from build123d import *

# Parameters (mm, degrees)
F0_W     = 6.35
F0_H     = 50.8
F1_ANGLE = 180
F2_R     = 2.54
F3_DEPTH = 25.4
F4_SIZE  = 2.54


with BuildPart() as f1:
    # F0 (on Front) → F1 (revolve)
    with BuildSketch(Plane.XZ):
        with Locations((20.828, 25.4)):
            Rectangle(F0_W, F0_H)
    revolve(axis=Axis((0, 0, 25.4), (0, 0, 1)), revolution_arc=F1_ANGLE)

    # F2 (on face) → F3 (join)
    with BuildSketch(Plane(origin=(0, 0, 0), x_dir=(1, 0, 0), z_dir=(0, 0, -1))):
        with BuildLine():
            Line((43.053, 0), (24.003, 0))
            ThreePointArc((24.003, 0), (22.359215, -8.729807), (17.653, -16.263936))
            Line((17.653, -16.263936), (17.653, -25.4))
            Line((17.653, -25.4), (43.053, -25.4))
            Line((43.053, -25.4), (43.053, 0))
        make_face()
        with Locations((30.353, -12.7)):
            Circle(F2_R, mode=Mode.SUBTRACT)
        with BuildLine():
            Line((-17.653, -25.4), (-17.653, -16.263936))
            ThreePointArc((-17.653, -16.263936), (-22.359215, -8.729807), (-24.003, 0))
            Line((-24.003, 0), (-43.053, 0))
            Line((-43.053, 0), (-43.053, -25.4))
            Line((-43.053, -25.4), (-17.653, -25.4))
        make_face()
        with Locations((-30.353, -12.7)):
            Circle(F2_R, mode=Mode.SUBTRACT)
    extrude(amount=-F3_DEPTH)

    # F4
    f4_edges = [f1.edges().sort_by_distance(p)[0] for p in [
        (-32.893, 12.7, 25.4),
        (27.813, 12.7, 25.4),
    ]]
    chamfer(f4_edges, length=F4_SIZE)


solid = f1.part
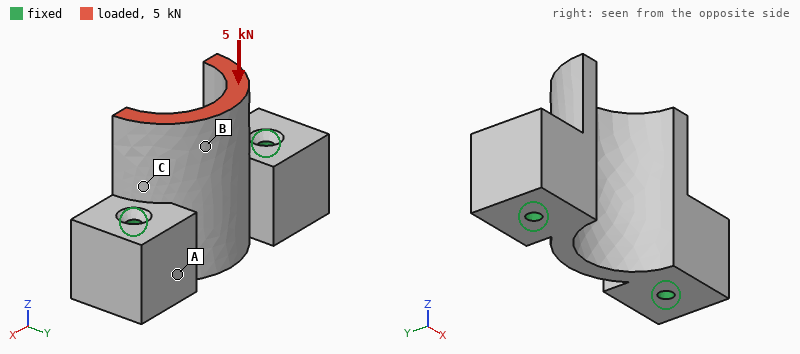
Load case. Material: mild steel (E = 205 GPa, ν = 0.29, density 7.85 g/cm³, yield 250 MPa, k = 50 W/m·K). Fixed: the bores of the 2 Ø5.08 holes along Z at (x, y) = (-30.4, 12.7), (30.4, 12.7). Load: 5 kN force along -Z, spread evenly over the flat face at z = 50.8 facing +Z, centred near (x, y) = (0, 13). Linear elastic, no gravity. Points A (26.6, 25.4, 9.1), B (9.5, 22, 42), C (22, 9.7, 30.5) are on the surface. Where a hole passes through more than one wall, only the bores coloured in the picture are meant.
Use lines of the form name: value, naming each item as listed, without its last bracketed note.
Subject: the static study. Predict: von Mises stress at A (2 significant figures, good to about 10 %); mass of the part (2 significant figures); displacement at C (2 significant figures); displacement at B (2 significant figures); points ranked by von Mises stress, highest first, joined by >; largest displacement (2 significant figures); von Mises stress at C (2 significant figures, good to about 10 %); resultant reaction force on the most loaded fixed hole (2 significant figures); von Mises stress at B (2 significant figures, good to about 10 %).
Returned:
von Mises stress at A: 4.7 MPa
mass of the part: 390 g
displacement at C: 2.3 µm
displacement at B: 5.9 µm
points ranked by von Mises stress, highest first, joined by >: C > B > A
largest displacement: 7.8 µm
von Mises stress at C: 20 MPa
resultant reaction force on the most loaded fixed hole: 2.5 kN
von Mises stress at B: 14 MPa
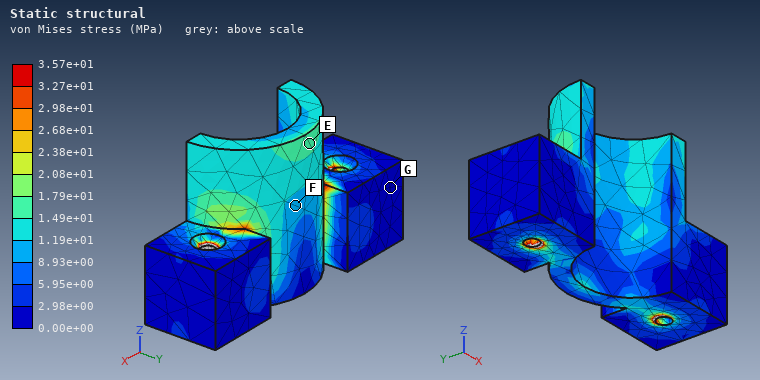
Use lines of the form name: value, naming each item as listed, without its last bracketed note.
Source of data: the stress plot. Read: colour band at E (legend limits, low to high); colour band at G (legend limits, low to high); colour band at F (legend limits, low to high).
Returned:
colour band at E: 1.49e+01 to 1.79e+01 MPa
colour band at G: 0.00e+00 to 2.98e+00 MPa
colour band at F: 8.93e+00 to 1.19e+01 MPa
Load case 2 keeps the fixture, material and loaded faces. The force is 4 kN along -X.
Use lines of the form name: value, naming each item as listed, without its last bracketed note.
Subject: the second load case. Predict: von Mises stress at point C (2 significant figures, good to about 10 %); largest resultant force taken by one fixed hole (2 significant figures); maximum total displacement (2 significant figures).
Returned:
von Mises stress at point C: 72 MPa
largest resultant force taken by one fixed hole: 3.3 kN
maximum total displacement: 47 µm
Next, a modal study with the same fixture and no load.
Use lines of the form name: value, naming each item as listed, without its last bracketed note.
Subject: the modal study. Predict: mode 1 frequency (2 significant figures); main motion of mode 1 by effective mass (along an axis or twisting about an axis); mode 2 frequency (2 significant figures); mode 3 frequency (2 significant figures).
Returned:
mode 1 frequency: 7700 Hz
main motion of mode 1 by effective mass: along Y
mode 2 frequency: 8800 Hz
mode 3 frequency: 12 kHz
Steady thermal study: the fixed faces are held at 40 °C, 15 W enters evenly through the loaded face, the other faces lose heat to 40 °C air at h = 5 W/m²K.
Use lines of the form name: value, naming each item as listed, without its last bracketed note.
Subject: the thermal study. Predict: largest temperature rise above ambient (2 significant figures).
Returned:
largest temperature rise above ambient: 28 K
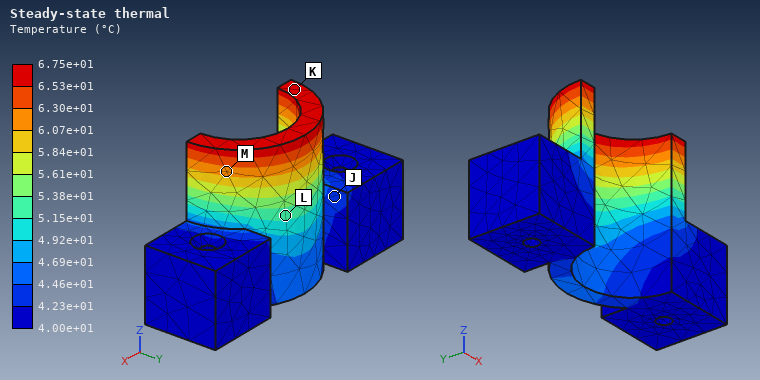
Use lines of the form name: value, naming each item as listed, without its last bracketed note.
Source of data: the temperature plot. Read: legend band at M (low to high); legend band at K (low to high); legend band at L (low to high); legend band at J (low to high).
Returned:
legend band at M: 6.07e+01 to 6.30e+01 °C
legend band at K: 6.53e+01 to 6.75e+01 °C
legend band at L: 5.15e+01 to 5.38e+01 °C
legend band at J: 4.23e+01 to 4.46e+01 °C
